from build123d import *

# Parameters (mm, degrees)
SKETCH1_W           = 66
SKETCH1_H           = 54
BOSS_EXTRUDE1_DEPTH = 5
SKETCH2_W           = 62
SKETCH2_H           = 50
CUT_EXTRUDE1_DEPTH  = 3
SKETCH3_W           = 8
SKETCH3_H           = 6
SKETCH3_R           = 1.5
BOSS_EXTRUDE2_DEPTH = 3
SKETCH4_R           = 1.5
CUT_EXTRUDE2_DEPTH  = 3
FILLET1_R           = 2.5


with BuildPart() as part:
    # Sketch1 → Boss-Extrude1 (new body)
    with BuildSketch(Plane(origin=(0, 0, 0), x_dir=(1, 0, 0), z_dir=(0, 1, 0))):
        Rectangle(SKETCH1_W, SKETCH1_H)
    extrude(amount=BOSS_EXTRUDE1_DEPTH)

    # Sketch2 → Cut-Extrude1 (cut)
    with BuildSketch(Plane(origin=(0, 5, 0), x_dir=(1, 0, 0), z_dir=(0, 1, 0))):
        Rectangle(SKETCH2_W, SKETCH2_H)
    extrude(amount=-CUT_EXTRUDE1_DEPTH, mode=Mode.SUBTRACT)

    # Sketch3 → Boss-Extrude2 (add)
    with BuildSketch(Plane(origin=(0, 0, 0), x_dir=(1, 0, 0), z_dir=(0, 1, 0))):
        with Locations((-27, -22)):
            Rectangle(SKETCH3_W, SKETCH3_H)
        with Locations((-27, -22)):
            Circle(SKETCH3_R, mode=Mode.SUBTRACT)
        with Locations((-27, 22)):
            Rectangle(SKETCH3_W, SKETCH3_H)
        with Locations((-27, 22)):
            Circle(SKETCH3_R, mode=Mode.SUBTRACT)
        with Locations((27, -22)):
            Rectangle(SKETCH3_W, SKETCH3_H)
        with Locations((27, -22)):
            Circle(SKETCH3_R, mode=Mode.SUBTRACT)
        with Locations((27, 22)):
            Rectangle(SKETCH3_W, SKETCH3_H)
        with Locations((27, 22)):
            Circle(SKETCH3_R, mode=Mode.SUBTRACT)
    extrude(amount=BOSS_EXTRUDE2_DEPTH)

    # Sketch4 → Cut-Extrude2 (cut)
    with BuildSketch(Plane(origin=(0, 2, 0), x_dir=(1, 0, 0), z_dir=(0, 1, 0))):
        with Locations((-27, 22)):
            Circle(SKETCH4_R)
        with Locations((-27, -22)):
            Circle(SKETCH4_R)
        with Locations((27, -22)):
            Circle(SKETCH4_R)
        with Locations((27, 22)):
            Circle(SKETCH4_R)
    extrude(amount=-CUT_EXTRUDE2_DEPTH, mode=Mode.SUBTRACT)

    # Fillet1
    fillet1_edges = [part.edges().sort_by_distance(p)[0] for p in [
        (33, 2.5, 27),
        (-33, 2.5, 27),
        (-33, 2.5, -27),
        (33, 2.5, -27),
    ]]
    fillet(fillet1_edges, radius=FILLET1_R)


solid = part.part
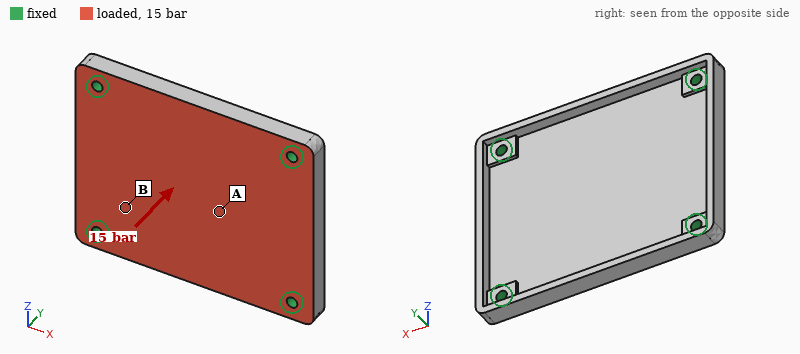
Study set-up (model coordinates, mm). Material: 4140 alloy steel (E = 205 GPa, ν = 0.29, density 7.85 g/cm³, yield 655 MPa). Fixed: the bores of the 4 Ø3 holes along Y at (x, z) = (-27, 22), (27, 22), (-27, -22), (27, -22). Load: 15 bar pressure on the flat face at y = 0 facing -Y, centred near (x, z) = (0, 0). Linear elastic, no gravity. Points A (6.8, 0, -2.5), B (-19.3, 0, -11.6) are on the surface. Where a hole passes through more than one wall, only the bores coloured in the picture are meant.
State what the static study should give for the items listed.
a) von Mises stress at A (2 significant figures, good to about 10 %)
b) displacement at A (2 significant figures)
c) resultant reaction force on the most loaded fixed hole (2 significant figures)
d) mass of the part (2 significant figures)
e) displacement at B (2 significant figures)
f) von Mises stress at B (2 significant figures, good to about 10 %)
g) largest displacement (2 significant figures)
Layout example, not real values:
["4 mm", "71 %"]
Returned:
["230 MPa", "0.26 mm", "1.4 kN", "68 g", "0.11 mm", "78 MPa", "0.28 mm"]
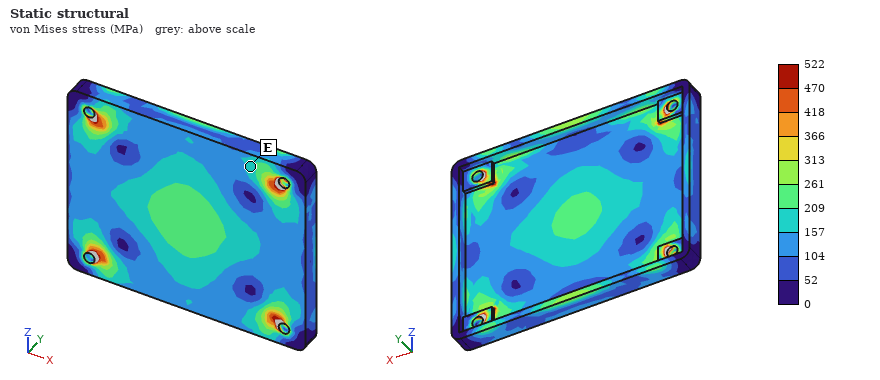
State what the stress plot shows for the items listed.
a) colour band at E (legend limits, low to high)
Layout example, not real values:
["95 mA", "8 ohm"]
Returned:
["157 to 209 MPa"]
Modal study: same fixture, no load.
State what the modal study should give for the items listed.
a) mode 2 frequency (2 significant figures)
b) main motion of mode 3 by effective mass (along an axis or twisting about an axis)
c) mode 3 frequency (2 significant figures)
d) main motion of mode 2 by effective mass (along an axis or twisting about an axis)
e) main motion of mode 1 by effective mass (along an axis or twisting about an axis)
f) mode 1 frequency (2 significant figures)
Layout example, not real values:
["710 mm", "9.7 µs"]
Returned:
["6400 Hz", "twisting about Z", "7400 Hz", "twisting about X", "along Y", "3700 Hz"]
